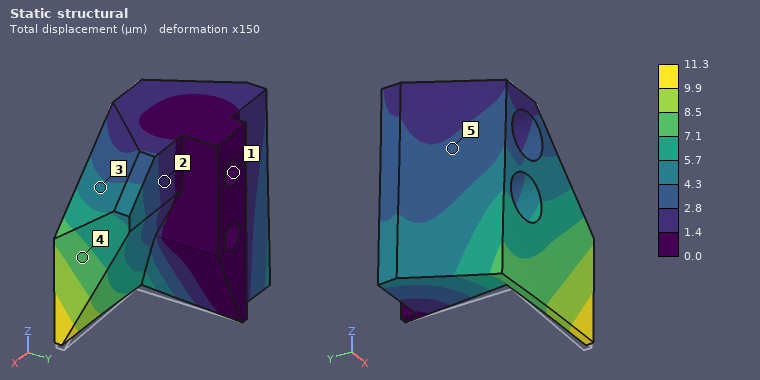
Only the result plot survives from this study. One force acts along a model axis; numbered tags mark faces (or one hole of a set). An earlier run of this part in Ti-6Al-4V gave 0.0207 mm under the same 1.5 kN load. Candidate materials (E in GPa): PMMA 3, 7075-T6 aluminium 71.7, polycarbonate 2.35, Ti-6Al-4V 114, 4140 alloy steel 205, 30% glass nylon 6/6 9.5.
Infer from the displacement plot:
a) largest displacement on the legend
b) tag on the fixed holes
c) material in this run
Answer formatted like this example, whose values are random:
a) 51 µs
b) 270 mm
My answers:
a) 11.3 µm
b) 1
c) 4140 alloy steel
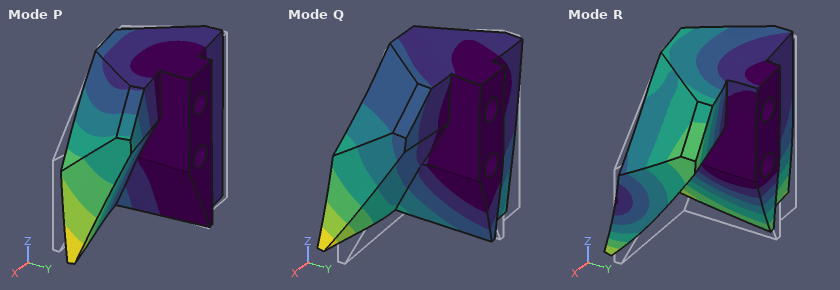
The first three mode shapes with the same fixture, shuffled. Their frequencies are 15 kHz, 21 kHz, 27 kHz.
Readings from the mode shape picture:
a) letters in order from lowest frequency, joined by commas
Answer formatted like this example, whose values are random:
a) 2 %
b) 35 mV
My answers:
a) P, Q, R
